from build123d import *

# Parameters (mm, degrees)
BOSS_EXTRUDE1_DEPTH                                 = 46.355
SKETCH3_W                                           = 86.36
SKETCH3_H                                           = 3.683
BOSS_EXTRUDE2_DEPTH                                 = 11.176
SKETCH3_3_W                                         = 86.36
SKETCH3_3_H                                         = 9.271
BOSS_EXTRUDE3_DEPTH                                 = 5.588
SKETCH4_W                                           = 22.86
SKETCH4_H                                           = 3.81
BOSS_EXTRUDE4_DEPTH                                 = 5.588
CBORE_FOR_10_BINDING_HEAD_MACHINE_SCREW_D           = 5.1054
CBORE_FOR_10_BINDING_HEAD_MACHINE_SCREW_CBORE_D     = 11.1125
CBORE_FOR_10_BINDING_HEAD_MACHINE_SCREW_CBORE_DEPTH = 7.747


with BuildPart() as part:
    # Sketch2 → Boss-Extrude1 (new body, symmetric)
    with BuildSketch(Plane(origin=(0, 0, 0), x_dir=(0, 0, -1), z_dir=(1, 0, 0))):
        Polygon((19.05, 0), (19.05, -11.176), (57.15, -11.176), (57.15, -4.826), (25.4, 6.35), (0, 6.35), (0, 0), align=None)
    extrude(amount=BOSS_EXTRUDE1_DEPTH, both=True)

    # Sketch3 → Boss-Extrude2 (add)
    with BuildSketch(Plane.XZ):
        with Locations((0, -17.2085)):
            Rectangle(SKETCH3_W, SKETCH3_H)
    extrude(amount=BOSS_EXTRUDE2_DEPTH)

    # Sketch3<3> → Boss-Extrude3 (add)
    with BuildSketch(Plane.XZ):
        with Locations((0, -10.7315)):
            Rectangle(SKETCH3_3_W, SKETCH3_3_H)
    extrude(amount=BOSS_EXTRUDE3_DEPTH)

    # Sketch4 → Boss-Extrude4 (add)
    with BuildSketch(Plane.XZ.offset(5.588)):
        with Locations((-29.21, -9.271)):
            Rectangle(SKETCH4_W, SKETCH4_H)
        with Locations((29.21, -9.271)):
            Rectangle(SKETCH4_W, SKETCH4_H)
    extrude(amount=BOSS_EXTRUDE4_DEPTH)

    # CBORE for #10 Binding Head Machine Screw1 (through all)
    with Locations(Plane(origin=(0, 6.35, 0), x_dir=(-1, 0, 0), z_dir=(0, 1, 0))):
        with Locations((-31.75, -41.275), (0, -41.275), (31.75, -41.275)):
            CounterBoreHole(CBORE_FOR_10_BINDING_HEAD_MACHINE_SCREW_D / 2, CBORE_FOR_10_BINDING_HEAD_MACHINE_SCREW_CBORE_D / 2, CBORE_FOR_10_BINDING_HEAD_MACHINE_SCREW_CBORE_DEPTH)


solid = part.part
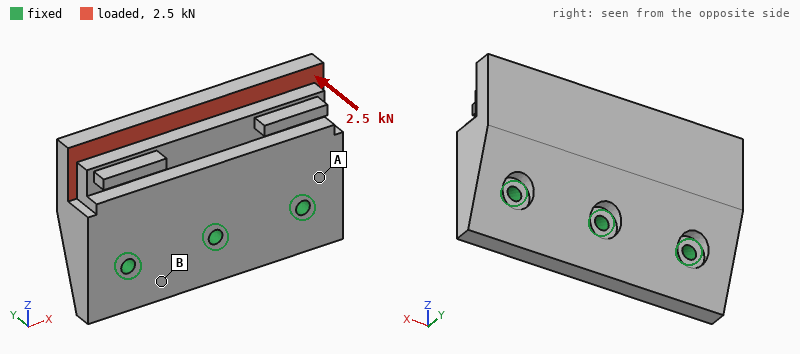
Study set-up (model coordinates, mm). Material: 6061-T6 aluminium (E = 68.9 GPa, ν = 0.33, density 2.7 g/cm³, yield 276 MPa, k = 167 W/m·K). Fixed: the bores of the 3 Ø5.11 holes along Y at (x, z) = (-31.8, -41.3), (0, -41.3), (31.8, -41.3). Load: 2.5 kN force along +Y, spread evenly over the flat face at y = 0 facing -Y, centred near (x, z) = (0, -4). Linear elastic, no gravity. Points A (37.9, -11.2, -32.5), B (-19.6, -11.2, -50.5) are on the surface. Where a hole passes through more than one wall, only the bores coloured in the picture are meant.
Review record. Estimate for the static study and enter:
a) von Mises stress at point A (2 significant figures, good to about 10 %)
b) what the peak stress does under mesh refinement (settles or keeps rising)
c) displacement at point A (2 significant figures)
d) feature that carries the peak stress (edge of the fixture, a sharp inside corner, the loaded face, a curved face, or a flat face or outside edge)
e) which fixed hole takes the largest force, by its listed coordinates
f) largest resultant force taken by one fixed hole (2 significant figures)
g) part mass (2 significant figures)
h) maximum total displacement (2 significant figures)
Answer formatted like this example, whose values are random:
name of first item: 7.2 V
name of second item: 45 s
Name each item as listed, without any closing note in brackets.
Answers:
von Mises stress at point A: 24 MPa
what the peak stress does under mesh refinement: keeps rising
displacement at point A: 13 µm
feature that carries the peak stress: edge of the fixture
which fixed hole takes the largest force, by its listed coordinates: (0, -41.3)
largest resultant force taken by one fixed hole: 900 N
part mass: 170 g
maximum total displacement: 80 µm
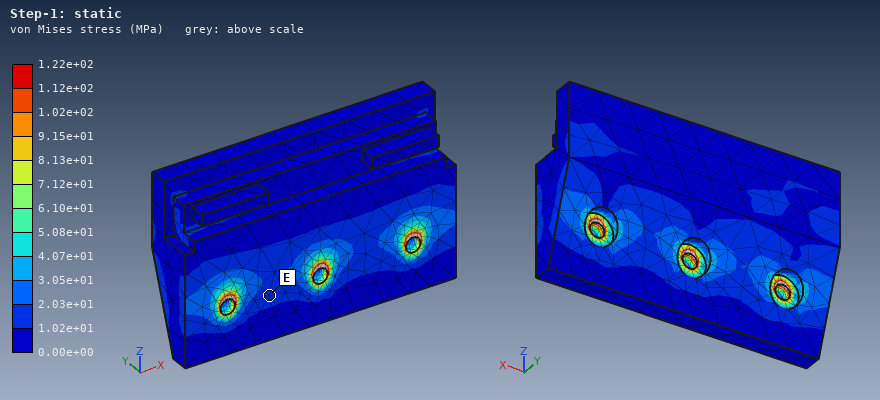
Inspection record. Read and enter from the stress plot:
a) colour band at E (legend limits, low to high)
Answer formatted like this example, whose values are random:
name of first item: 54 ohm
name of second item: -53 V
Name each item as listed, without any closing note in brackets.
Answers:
colour band at E: 1.02e+01 to 2.03e+01 MPa
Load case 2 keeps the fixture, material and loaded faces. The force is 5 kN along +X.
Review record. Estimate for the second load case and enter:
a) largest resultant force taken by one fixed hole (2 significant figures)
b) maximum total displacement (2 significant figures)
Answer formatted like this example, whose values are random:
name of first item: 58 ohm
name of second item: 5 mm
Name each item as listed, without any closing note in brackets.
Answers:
largest resultant force taken by one fixed hole: 3.2 kN
maximum total displacement: 21 µm
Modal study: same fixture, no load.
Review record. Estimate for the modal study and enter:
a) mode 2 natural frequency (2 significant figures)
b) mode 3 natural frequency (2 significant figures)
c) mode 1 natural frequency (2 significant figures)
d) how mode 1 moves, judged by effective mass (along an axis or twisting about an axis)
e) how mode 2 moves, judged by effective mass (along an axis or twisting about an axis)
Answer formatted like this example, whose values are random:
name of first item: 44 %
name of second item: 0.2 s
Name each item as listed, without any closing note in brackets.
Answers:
mode 2 natural frequency: 7200 Hz
mode 3 natural frequency: 13 kHz
mode 1 natural frequency: 4500 Hz
how mode 1 moves, judged by effective mass: along Y
how mode 2 moves, judged by effective mass: twisting about Z
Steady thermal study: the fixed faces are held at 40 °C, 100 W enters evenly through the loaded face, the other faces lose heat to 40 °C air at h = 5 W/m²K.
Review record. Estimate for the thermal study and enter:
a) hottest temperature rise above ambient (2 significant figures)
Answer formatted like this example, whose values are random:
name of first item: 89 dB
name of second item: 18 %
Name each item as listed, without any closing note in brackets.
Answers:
hottest temperature rise above ambient: 27 K
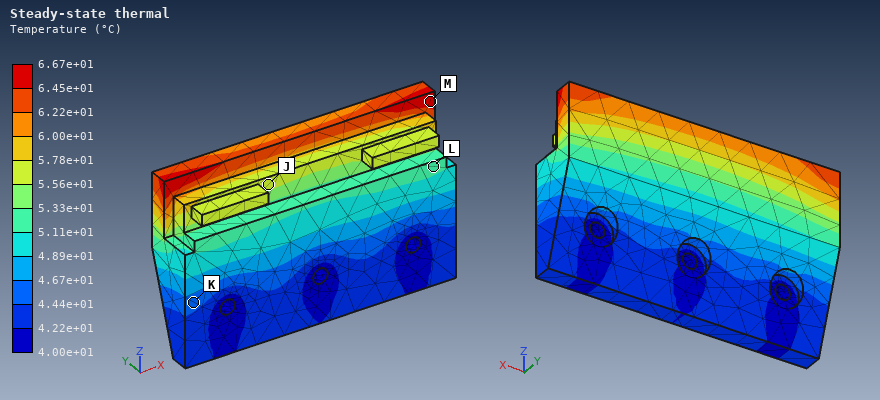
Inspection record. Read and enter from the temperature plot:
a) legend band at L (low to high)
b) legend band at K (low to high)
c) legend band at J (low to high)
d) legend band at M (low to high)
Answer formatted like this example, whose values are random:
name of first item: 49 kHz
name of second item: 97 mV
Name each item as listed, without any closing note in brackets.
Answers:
legend band at L: 5.11e+01 to 5.33e+01 °C
legend band at K: 4.44e+01 to 4.67e+01 °C
legend band at J: 5.56e+01 to 5.78e+01 °C
legend band at M: 6.45e+01 to 6.67e+01 °C
